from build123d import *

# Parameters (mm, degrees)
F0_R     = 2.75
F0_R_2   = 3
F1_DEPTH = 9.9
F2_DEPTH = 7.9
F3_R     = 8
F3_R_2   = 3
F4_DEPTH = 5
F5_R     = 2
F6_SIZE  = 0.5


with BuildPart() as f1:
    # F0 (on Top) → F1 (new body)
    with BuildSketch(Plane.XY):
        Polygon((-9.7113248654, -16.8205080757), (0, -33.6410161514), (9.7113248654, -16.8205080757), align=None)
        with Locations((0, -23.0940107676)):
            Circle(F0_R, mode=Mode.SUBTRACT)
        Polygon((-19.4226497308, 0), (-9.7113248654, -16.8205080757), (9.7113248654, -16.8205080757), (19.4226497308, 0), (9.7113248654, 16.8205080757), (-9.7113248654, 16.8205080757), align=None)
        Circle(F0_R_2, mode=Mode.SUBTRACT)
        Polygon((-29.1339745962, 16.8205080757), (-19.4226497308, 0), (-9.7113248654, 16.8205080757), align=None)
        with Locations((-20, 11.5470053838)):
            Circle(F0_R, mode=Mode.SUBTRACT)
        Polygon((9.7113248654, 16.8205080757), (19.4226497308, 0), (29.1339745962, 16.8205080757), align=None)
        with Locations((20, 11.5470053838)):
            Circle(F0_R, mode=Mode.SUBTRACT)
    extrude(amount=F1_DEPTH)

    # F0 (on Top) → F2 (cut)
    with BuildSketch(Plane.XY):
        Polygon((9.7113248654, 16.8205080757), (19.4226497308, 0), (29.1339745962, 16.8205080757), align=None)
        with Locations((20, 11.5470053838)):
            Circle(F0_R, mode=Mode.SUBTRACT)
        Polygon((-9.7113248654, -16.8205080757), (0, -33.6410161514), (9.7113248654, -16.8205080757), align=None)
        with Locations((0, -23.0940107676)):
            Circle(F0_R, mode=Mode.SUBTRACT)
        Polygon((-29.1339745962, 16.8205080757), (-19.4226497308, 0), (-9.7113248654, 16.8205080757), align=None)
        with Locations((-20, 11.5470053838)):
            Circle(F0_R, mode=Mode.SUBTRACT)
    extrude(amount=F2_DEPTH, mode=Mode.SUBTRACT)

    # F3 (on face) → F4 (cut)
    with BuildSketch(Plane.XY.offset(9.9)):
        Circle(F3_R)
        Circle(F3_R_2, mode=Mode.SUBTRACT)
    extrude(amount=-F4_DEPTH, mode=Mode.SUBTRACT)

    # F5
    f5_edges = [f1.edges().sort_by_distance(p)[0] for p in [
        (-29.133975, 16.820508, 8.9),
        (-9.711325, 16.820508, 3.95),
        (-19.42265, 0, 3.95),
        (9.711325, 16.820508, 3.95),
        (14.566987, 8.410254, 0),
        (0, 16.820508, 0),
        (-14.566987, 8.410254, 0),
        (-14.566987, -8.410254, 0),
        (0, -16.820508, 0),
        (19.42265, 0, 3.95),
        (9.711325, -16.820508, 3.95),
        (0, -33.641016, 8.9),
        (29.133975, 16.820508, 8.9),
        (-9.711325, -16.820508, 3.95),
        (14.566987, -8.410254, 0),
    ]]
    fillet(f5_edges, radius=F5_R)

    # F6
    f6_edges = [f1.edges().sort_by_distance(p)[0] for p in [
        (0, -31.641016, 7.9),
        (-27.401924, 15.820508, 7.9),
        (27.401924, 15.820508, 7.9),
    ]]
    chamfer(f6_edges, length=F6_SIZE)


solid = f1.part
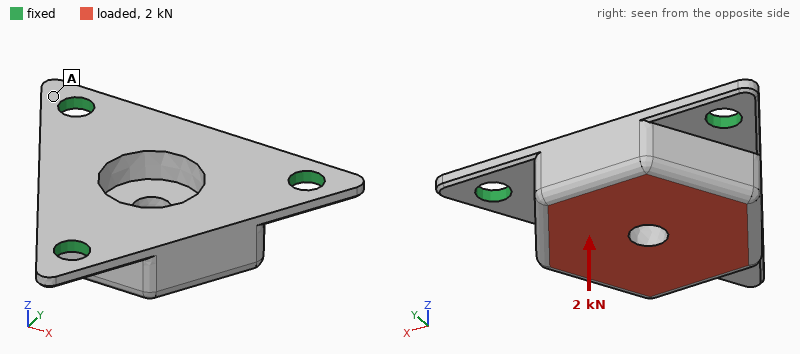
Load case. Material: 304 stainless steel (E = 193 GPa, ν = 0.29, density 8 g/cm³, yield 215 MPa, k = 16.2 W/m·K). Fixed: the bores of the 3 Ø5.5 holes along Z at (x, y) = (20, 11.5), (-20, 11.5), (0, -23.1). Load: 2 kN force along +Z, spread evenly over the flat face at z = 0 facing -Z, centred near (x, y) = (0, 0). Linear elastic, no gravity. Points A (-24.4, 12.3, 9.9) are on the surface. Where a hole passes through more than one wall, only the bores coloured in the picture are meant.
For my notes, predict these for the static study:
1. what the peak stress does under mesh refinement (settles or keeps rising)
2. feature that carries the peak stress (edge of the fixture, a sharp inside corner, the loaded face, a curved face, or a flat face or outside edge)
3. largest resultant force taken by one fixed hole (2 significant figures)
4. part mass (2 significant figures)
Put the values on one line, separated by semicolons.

keeps rising; edge of the fixture; 840 N; 74 g
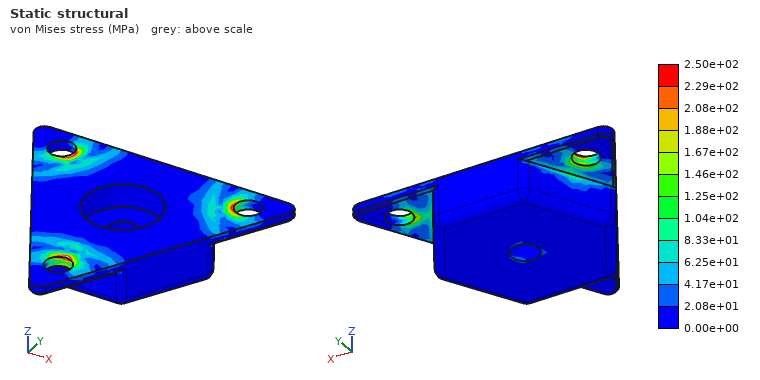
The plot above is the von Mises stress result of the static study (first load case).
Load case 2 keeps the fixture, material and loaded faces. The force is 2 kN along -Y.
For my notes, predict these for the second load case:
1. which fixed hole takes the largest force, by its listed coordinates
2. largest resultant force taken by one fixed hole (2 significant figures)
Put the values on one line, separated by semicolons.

(0, -23.1); 1.2 kN
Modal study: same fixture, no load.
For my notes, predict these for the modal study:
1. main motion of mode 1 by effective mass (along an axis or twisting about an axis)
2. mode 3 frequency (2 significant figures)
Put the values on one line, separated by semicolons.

along Z; 12 kHz
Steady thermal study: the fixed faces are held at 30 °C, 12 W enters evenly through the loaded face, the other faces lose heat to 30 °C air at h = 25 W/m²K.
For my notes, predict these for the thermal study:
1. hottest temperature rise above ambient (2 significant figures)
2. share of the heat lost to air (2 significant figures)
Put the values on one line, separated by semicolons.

54 K; 26 %
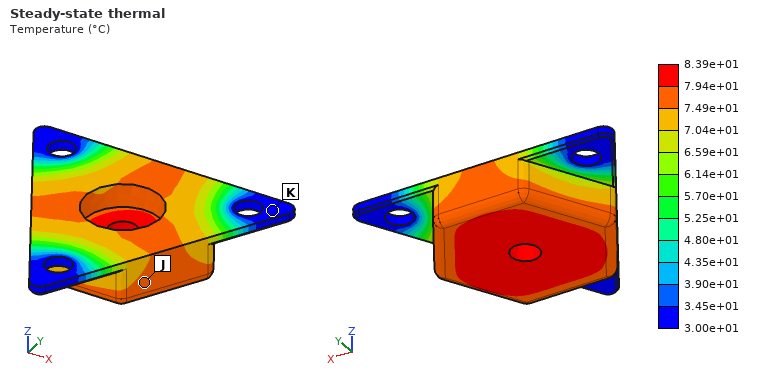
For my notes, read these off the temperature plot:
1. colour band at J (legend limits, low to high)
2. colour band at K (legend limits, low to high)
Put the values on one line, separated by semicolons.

7.49e+01 to 7.94e+01 °C; 3.00e+01 to 3.45e+01 °C
